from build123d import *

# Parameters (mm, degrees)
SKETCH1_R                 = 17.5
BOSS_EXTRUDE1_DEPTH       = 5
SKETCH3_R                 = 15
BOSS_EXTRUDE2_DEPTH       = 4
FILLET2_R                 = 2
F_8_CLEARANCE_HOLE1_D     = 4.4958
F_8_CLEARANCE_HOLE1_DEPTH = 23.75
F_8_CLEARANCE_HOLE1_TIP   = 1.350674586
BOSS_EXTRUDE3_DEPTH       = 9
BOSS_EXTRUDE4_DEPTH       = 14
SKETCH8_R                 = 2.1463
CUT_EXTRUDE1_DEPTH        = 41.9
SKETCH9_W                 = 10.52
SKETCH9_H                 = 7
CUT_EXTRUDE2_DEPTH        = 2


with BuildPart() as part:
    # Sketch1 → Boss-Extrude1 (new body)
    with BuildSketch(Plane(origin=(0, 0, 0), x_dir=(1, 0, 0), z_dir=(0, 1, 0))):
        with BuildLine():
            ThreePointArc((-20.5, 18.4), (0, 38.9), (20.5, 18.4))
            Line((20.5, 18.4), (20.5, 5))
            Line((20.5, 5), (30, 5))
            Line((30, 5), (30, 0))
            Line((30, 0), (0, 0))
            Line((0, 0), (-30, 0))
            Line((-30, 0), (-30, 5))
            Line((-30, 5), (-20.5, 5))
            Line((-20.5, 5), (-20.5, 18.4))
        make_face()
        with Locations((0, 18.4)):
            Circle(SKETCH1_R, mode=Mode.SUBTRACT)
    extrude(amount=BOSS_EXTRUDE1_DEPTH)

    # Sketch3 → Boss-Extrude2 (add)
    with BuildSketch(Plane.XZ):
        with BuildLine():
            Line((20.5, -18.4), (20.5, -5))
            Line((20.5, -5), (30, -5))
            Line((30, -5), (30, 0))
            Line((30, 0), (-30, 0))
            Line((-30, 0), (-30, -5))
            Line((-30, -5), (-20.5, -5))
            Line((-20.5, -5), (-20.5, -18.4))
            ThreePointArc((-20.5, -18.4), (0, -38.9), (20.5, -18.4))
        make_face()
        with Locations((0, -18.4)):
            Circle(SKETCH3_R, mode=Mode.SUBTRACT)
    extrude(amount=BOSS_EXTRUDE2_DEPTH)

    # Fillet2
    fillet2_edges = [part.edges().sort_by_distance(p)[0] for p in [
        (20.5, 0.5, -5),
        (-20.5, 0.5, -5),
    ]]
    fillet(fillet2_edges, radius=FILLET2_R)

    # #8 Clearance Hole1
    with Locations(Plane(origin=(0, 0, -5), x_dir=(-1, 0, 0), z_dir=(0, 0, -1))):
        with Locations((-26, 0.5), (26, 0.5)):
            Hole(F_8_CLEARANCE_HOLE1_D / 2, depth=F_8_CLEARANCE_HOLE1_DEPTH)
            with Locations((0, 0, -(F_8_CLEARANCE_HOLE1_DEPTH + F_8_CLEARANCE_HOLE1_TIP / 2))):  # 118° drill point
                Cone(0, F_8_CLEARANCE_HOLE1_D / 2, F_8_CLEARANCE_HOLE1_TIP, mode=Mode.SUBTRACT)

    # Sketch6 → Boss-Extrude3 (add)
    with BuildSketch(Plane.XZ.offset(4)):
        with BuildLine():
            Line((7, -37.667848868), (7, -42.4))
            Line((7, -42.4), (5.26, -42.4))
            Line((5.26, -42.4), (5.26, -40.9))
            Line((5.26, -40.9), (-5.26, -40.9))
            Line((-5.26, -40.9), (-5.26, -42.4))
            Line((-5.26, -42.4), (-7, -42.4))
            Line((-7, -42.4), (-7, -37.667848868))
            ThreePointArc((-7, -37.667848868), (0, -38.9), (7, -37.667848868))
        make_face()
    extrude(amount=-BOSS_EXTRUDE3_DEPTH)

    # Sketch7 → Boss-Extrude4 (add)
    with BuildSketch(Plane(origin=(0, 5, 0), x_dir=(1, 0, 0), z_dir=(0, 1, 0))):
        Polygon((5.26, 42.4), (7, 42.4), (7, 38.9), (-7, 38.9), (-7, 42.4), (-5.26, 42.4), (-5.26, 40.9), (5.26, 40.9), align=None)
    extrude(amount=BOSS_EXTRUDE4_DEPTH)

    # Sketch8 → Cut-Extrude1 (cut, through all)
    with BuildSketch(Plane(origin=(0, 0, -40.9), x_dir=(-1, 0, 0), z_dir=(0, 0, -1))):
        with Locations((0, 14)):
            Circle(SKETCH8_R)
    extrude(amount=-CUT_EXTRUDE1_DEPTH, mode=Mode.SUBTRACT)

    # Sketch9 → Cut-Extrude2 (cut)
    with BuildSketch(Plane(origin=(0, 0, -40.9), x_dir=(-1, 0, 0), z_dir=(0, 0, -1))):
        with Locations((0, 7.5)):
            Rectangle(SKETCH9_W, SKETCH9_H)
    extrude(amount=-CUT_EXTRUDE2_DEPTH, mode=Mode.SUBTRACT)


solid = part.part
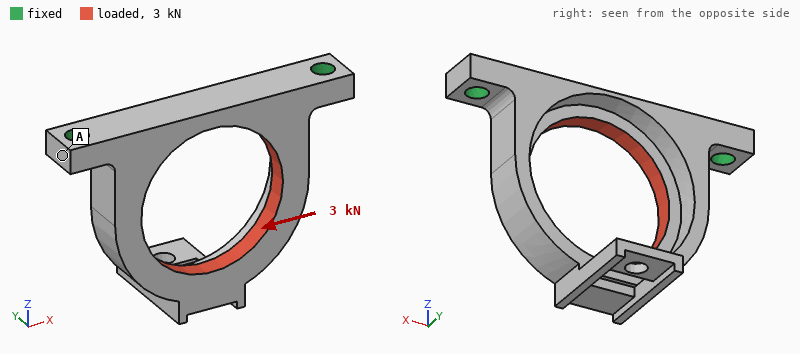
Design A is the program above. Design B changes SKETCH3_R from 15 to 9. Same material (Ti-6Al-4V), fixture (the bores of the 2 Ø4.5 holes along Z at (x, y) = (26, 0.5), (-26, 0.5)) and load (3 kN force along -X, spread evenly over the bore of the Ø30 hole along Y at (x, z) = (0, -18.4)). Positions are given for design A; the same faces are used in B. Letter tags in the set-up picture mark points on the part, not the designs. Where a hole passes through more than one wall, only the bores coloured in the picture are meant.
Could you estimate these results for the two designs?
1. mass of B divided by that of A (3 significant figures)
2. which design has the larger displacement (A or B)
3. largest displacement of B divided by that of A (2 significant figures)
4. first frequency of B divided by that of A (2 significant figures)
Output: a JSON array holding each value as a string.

["1.28", "A", "0.31", "0.96"]
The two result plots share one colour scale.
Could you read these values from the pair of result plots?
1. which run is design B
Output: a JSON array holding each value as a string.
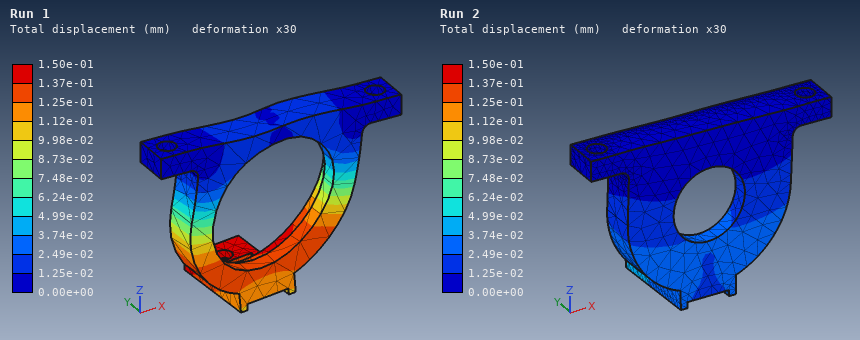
["Run 2"]
